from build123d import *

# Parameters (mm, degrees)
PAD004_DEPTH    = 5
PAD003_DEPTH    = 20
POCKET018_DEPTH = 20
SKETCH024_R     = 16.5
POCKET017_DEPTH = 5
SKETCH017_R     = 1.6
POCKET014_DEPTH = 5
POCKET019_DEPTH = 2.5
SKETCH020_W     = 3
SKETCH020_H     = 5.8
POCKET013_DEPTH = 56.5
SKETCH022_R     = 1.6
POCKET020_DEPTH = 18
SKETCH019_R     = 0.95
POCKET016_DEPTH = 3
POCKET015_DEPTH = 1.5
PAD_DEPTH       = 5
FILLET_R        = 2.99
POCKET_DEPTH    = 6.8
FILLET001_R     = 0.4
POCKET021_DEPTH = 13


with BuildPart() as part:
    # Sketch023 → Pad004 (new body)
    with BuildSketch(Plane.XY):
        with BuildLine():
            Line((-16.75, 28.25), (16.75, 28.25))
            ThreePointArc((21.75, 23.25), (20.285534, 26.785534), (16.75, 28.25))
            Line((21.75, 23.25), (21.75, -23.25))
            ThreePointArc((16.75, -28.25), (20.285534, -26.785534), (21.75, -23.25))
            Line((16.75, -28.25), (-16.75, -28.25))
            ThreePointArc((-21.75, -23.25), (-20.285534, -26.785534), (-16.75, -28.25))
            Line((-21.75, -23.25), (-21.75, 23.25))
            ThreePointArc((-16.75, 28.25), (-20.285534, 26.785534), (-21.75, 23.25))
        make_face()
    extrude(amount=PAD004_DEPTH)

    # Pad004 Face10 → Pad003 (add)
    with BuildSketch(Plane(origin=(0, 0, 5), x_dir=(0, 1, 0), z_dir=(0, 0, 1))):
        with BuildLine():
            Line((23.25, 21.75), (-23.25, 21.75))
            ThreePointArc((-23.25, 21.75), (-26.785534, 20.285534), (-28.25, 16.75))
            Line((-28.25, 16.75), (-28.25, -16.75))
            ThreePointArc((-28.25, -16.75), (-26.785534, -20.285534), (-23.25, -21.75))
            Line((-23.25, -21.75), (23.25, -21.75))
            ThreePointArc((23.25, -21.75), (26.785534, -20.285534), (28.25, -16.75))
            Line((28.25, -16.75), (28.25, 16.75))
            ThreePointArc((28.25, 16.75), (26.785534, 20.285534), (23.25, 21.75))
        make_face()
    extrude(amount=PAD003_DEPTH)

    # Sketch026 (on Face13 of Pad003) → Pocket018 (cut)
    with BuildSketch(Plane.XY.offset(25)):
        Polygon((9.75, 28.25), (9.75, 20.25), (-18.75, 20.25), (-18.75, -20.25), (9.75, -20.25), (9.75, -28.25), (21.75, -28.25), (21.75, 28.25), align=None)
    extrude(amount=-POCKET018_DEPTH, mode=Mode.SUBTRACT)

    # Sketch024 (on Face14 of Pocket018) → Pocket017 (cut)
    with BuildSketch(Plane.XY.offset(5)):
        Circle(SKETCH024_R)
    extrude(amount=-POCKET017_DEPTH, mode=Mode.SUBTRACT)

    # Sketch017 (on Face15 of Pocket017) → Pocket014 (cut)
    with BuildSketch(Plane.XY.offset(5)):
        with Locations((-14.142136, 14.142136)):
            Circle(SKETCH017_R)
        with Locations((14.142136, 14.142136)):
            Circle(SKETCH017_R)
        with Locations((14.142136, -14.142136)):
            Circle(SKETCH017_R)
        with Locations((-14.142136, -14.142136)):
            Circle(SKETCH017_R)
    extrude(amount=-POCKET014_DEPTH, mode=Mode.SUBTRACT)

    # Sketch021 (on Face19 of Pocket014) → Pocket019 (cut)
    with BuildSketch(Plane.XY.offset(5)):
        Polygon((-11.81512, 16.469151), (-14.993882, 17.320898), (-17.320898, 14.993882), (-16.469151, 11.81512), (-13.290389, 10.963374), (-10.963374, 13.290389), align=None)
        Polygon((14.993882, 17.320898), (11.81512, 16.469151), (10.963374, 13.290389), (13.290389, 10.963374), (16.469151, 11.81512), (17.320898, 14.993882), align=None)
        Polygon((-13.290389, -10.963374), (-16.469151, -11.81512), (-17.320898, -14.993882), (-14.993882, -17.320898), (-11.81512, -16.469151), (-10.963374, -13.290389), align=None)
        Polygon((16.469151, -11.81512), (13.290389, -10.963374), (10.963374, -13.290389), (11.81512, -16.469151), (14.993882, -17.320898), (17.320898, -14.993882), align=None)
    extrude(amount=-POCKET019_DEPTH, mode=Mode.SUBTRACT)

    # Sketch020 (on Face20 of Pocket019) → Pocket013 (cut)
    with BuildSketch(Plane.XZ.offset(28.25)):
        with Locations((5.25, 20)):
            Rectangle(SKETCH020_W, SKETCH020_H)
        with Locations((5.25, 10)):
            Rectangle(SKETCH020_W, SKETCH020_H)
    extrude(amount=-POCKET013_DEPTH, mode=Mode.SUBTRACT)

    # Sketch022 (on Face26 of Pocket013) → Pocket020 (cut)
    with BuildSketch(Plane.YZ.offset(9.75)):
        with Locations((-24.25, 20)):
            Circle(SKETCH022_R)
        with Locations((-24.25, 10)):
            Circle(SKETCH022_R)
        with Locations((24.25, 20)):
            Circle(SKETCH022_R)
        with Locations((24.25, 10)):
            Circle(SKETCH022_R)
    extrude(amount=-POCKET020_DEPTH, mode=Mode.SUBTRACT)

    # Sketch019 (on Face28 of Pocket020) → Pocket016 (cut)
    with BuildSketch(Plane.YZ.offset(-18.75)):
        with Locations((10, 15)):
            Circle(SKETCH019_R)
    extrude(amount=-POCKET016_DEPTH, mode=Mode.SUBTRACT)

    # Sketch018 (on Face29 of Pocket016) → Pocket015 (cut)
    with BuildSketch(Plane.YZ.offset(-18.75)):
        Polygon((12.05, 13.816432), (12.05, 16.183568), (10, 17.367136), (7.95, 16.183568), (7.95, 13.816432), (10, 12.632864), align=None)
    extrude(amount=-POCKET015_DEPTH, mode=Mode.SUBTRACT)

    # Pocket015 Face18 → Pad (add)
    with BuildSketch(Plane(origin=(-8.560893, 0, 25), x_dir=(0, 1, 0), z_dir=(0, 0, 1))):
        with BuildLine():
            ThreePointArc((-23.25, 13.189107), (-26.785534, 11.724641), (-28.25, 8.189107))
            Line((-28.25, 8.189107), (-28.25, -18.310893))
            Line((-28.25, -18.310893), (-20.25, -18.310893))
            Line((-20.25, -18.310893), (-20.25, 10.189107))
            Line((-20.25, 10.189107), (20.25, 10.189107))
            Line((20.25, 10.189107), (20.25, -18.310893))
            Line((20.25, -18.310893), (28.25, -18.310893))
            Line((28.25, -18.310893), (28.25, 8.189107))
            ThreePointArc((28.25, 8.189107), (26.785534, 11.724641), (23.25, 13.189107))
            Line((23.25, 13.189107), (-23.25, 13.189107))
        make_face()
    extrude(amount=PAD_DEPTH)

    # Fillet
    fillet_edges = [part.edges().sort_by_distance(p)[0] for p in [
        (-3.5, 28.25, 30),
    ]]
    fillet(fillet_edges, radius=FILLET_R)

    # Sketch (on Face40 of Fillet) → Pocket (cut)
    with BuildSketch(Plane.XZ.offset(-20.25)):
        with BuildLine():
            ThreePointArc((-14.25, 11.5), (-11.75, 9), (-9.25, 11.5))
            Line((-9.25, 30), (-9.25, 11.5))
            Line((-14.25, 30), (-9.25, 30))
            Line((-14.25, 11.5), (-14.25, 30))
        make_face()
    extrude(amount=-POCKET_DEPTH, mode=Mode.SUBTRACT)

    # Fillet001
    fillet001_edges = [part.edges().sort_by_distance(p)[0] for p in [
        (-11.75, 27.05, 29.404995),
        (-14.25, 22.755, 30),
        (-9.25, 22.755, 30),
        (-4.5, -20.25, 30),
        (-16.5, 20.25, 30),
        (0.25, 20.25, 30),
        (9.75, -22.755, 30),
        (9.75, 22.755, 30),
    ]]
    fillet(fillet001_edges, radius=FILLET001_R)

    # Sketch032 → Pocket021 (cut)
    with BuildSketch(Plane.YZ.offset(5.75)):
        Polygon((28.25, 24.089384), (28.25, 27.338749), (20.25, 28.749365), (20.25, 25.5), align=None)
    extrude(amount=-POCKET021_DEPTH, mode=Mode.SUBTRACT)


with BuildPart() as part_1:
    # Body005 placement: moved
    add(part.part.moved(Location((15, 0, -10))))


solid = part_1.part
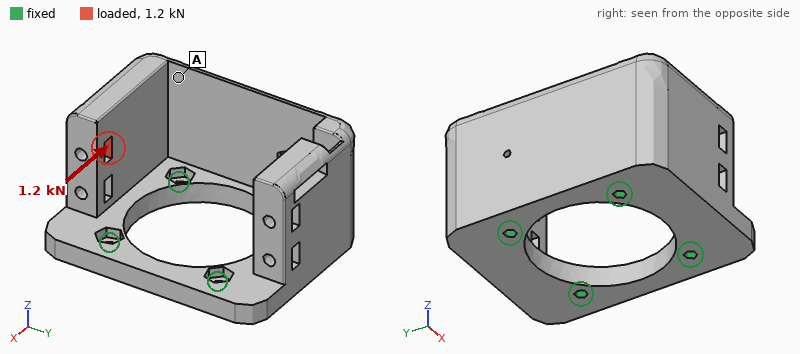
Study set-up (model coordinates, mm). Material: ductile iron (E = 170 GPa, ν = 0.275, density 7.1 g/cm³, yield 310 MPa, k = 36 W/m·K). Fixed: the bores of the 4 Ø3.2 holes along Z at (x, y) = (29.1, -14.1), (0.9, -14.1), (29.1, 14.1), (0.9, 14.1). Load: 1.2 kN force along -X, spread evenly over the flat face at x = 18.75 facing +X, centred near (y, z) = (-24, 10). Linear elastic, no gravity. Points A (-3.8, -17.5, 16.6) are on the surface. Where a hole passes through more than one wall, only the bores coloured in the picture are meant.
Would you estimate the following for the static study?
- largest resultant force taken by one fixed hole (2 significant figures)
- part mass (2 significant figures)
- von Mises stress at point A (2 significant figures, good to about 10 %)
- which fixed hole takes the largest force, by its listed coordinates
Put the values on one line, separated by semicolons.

1.1 kN; 150 g; 14 MPa; (29.1, -14.1)
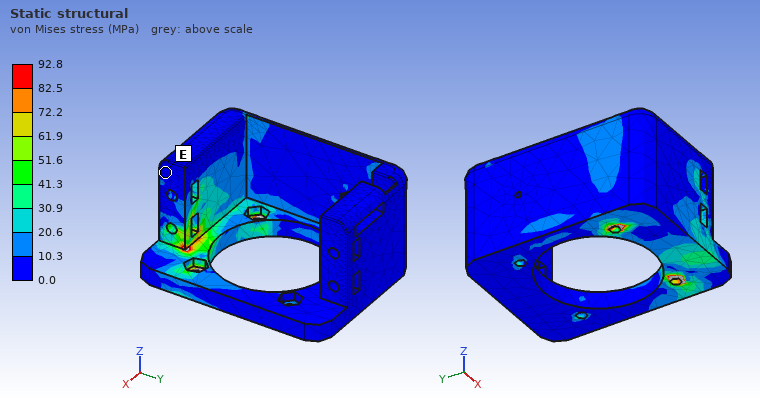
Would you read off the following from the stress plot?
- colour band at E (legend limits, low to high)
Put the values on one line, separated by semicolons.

0.0 to 10.3 MPa
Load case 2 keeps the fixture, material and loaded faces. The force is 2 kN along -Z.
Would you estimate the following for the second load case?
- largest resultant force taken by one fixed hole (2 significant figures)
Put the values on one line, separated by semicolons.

1.3 kN
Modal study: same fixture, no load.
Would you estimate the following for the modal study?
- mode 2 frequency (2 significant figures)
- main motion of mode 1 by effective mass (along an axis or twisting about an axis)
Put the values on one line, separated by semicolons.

4900 Hz; along Y
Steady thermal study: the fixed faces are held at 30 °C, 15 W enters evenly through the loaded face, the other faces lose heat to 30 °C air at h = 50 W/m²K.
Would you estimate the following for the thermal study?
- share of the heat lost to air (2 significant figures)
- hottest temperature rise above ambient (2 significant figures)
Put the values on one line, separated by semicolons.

44 %; 75 K
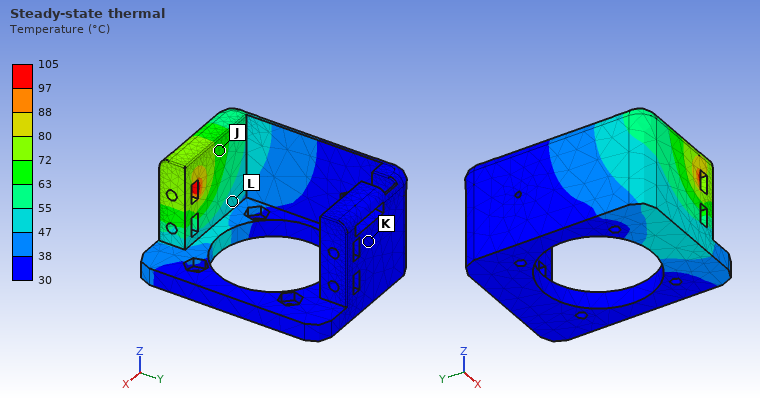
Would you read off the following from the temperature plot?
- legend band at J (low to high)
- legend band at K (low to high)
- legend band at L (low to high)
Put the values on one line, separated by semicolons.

63 to 72 °C; 30 to 38 °C; 47 to 55 °C
